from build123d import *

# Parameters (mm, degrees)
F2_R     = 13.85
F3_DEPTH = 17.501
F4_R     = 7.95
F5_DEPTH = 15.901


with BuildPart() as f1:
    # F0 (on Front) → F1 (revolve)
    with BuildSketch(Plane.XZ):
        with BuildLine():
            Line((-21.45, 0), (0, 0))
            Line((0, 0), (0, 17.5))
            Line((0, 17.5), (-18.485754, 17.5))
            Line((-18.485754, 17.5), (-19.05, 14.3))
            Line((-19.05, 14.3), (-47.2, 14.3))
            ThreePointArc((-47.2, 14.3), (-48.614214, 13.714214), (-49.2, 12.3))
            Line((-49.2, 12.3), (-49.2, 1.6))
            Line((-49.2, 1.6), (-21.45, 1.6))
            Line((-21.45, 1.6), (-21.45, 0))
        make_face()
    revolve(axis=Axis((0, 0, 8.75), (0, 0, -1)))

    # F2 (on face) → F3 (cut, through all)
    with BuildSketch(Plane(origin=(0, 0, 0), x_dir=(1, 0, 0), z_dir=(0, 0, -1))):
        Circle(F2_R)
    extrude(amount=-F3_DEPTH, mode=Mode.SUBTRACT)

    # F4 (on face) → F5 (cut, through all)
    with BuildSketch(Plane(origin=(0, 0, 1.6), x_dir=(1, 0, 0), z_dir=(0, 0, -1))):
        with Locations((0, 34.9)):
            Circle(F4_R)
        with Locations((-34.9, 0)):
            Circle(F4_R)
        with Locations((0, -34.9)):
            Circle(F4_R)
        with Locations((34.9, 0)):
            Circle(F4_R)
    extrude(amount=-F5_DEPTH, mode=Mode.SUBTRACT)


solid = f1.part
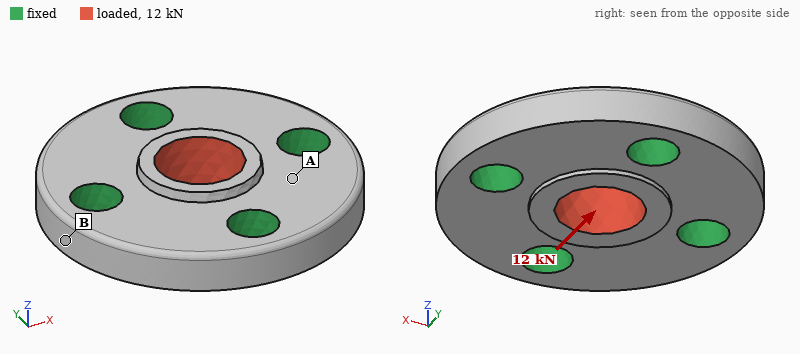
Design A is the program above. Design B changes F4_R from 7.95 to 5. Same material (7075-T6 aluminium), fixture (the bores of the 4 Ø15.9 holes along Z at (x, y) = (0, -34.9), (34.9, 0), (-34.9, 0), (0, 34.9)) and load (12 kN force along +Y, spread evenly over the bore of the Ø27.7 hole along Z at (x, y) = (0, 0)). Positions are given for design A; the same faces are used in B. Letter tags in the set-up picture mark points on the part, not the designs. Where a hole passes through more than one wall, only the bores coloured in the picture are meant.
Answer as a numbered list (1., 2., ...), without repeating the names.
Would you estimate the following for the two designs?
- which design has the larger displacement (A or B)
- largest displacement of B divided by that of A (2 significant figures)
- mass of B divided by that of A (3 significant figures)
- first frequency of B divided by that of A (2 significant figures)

1. B
2. 1.2
3. 1.07
4. 0.77
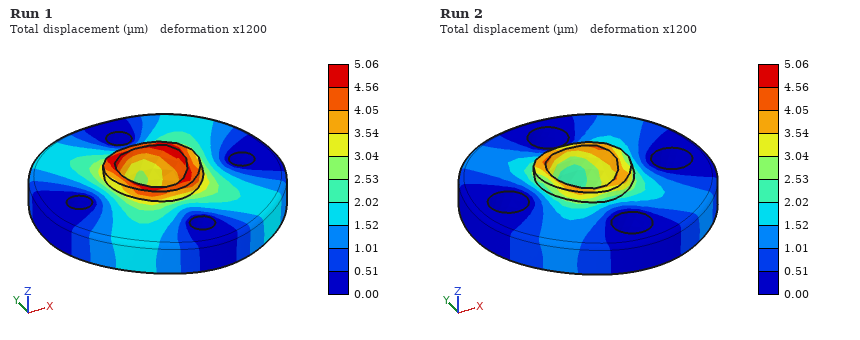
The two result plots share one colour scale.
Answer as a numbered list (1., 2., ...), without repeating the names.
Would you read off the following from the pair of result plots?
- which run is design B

1. Run 1
